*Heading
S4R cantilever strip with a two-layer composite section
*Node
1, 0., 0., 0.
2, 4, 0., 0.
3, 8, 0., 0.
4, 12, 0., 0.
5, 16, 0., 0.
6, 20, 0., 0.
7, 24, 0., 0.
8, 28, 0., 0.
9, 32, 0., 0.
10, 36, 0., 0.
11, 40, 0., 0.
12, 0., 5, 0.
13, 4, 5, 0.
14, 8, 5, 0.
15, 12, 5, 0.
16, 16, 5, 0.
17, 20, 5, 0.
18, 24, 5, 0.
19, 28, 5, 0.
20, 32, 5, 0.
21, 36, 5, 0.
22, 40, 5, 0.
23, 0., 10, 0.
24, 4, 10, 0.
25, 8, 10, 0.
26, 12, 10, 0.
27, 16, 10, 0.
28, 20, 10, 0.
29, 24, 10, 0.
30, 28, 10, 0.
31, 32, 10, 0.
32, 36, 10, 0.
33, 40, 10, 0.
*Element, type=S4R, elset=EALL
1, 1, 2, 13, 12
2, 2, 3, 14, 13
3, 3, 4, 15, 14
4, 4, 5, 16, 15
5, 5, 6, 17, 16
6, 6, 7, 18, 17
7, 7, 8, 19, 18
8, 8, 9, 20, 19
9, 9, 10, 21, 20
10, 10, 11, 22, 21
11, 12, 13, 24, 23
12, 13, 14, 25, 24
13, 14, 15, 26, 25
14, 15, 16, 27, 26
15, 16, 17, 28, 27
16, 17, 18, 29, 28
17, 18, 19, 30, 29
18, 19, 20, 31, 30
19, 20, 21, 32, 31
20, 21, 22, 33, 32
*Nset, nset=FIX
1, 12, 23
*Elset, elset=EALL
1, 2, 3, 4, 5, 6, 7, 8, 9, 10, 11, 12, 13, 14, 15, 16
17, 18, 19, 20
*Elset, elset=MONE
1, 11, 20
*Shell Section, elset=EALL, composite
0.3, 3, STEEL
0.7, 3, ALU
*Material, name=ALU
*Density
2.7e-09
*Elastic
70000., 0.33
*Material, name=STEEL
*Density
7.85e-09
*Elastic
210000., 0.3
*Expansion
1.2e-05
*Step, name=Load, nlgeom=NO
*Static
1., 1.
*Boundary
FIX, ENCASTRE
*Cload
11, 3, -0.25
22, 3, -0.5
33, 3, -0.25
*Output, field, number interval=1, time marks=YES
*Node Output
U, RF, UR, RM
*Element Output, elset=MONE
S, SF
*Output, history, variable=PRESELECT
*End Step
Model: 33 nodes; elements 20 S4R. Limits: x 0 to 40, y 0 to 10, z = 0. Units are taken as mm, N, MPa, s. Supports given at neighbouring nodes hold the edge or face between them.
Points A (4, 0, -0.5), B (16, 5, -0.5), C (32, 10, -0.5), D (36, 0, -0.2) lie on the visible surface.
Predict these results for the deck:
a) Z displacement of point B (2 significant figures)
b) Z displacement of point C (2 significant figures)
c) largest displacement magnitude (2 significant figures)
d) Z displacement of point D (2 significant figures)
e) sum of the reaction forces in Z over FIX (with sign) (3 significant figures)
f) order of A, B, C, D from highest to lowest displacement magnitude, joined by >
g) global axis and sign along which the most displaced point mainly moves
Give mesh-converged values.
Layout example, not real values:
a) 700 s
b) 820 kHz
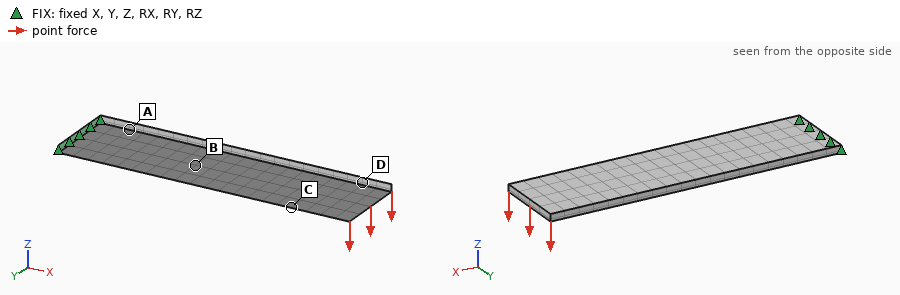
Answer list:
a) -0.045 mm
b) -0.15 mm
c) 0.22 mm
d) -0.19 mm
e) 1.00 N
f) D > C > B > A
g) -Z
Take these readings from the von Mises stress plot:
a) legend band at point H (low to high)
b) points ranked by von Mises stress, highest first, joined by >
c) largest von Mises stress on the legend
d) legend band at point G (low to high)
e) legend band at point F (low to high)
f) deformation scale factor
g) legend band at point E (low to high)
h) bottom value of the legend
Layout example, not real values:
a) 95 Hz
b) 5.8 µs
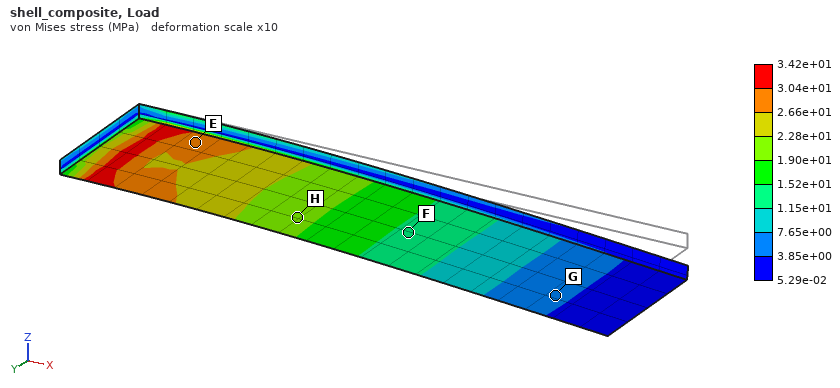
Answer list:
a) 1.90e+01 to 2.28e+01 MPa
b) E > H > F > G
c) 3.42e+01 MPa
d) 3.85e+00 to 7.65e+00 MPa
e) 1.15e+01 to 1.52e+01 MPa
f) 10
g) 2.66e+01 to 3.04e+01 MPa
h) 5.29e-02 MPa
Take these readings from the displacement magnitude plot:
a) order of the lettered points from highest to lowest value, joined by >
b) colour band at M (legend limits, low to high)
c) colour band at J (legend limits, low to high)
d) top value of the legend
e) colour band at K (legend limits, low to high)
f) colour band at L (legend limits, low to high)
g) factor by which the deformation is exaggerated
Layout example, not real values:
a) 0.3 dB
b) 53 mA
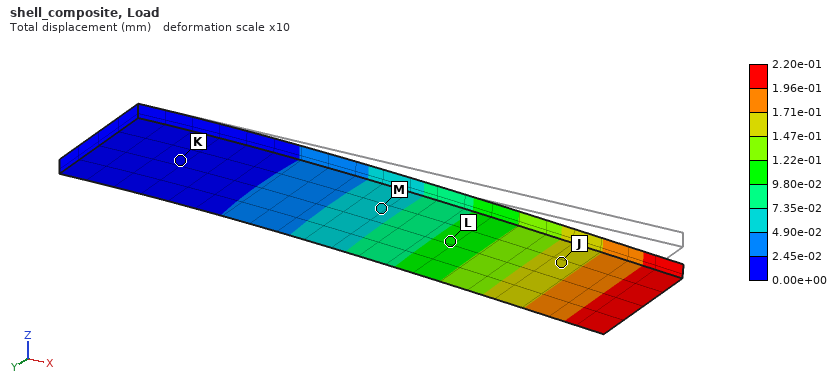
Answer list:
a) J > L > M > K
b) 4.90e-02 to 7.35e-02 mm
c) 1.47e-01 to 1.71e-01 mm
d) 2.20e-01 mm
e) 0.00e+00 to 2.45e-02 mm
f) 9.80e-02 to 1.22e-01 mm
g) 10
